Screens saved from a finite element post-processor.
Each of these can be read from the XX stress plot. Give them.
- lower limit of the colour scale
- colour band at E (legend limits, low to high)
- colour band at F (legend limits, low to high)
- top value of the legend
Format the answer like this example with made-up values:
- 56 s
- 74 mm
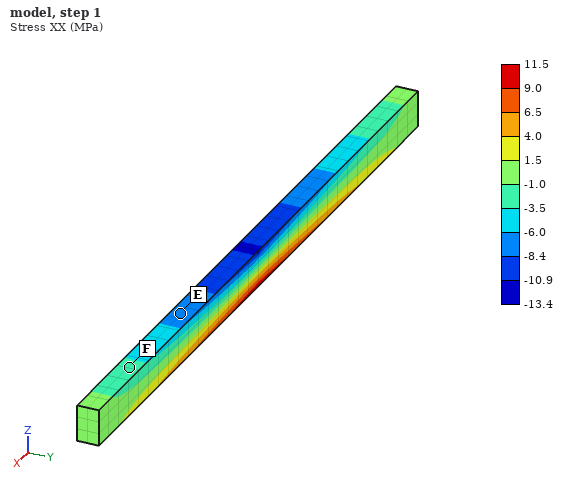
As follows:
- -13.4 MPa
- -8.4 to -6.0 MPa
- -3.5 to -1.0 MPa
- 11.5 MPa
